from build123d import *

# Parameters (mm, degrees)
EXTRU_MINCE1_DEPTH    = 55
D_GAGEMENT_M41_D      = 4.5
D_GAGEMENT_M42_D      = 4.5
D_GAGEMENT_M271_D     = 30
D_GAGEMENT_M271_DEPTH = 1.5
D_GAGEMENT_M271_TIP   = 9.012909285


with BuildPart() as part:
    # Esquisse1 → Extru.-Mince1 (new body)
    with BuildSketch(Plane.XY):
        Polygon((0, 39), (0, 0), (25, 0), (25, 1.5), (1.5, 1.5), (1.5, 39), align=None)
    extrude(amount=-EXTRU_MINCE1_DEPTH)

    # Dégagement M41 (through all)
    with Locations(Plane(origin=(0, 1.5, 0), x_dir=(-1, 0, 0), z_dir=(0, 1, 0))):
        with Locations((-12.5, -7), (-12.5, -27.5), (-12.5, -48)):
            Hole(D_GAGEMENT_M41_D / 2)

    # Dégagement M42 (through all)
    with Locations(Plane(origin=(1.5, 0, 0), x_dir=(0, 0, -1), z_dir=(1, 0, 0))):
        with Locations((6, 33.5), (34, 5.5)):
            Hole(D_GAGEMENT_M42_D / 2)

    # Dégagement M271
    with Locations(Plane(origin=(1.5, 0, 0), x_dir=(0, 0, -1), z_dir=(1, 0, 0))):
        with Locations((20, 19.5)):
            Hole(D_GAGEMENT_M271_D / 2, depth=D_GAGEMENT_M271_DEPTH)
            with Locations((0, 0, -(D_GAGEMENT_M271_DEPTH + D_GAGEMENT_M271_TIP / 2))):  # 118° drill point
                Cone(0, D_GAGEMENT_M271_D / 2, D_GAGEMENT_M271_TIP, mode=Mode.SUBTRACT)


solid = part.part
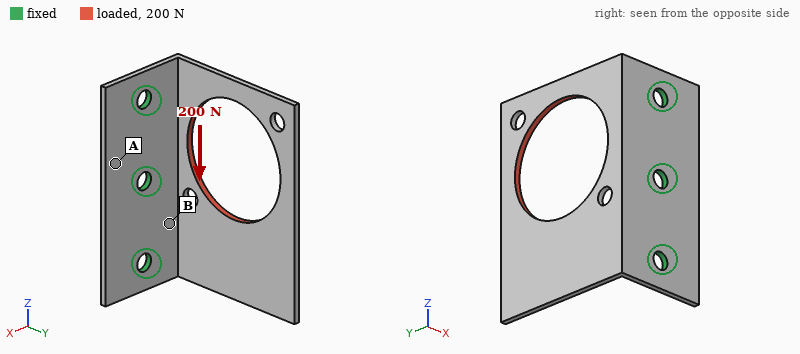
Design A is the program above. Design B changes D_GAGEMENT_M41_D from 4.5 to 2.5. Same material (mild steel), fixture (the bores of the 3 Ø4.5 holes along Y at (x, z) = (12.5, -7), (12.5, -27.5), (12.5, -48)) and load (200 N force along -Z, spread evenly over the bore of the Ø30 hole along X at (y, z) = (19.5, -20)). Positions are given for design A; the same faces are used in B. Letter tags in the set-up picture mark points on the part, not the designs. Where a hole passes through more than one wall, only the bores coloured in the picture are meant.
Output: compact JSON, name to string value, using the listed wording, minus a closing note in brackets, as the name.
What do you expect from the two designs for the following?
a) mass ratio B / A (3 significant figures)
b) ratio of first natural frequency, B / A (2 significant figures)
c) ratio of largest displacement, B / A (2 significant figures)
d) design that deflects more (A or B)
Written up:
{"mass ratio B / A": "1.01", "ratio of first natural frequency, B / A": "0.97", "ratio of largest displacement, B / A": "1.2", "design that deflects more": "B"}
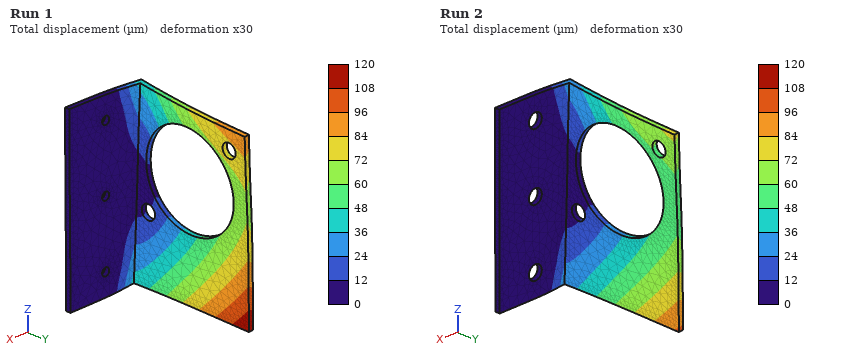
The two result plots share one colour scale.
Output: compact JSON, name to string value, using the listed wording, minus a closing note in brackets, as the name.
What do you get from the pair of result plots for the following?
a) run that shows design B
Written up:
{"run that shows design B": "Run 1"}
